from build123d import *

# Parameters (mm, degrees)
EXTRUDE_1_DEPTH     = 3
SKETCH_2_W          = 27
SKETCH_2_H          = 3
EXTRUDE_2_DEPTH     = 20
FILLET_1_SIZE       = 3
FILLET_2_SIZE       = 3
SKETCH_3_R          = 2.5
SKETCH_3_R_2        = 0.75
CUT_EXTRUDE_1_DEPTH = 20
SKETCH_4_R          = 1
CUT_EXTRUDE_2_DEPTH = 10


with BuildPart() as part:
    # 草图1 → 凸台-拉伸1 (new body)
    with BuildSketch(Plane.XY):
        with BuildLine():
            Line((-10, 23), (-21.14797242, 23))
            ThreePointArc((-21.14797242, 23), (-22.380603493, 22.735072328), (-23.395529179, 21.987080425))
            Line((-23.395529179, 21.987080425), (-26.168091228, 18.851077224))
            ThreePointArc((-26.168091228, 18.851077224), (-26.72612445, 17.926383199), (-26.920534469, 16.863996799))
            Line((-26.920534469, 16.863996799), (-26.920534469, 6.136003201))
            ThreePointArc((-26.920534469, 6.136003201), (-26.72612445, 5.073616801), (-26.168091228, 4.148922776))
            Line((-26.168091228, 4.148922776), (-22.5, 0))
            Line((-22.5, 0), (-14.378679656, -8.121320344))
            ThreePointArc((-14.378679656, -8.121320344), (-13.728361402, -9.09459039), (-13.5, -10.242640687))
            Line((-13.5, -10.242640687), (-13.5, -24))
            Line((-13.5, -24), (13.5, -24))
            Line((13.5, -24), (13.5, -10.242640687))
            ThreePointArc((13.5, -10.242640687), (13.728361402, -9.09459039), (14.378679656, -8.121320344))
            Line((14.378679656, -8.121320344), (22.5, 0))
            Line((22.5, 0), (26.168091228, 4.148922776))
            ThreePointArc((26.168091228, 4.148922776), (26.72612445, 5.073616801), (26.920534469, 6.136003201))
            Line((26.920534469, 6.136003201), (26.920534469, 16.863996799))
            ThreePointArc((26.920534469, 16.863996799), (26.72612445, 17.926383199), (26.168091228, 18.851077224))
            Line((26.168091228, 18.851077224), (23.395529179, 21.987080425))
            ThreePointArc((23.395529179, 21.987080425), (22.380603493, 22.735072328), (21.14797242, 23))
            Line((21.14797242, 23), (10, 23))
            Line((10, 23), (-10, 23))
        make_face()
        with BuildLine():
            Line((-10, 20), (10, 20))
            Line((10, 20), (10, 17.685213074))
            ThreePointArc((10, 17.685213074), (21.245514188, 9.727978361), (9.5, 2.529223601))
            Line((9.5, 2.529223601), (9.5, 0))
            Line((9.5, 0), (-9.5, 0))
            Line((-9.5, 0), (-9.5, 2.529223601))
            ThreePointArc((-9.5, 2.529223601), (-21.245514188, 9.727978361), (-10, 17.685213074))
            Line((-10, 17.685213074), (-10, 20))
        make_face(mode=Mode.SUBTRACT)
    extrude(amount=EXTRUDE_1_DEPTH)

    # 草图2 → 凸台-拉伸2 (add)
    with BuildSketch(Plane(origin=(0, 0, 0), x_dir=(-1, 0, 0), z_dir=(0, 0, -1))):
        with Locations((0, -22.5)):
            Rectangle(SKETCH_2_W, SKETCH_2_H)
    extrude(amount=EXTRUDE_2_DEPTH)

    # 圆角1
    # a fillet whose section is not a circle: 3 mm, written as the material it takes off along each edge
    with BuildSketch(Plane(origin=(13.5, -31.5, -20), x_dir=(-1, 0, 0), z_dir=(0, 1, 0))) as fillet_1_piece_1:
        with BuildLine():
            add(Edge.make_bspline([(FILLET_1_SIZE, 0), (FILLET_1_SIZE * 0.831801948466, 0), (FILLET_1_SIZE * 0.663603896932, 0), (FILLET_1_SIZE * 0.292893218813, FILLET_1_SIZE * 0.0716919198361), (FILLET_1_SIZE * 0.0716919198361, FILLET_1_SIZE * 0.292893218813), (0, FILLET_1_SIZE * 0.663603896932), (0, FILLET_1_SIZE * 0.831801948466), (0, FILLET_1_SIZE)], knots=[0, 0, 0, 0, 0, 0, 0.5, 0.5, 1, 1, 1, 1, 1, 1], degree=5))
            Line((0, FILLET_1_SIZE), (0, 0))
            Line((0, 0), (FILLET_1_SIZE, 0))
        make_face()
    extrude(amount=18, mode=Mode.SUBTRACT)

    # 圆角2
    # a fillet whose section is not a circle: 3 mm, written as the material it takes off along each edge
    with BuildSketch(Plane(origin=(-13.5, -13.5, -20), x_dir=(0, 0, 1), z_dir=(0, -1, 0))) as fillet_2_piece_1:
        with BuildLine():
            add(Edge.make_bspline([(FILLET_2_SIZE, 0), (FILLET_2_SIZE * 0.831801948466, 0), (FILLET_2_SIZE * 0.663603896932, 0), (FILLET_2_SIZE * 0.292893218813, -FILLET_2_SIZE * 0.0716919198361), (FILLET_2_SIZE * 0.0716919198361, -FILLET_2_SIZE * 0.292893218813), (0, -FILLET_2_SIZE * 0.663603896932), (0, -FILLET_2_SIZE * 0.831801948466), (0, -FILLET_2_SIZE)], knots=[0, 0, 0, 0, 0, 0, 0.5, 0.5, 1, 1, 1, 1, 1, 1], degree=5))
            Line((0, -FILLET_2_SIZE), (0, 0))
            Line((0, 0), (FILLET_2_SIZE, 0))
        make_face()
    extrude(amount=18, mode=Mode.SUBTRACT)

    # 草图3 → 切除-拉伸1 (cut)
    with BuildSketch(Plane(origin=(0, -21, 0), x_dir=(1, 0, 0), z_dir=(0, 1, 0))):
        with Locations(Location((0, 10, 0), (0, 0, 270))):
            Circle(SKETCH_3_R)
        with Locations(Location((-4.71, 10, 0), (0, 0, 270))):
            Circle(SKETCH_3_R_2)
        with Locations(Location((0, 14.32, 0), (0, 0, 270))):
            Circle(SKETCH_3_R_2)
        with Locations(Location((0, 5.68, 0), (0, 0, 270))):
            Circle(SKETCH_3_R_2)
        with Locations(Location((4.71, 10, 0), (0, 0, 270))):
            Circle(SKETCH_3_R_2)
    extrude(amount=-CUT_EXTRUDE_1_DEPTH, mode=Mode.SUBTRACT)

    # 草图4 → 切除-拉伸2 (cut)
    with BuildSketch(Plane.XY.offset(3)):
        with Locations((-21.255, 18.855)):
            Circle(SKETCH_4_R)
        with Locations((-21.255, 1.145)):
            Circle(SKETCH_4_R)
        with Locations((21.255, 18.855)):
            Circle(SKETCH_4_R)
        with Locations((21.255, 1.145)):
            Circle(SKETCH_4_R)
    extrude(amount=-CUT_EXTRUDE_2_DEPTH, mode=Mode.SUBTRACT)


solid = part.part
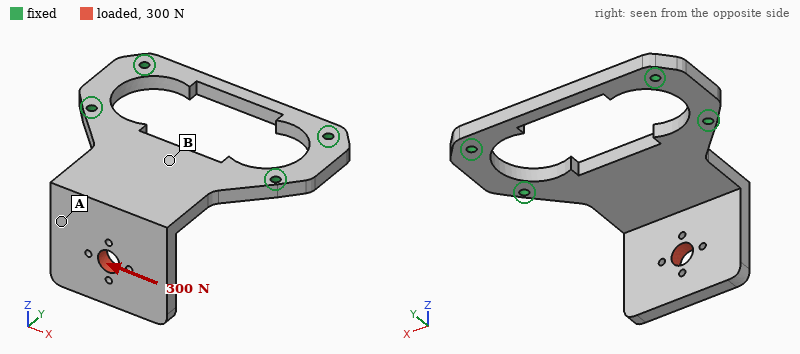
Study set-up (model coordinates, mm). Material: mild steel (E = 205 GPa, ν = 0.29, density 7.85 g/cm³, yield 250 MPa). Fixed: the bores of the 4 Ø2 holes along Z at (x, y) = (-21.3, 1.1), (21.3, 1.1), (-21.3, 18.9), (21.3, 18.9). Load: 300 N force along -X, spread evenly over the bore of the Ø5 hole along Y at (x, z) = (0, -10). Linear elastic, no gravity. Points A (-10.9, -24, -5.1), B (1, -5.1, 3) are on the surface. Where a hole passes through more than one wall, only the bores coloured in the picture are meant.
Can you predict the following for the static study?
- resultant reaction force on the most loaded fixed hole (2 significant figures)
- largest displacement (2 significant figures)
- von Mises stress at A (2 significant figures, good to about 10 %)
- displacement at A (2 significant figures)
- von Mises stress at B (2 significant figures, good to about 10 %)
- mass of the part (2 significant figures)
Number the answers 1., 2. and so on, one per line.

1. 260 N
2. 73 µm
3. 15 MPa
4. 38 µm
5. 43 MPa
6. 40 g
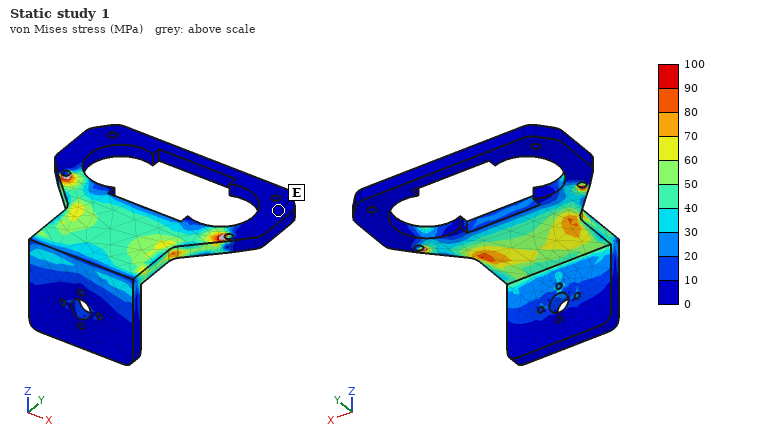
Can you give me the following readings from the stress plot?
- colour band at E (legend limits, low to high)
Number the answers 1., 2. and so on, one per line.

1. 0 to 10 MPa
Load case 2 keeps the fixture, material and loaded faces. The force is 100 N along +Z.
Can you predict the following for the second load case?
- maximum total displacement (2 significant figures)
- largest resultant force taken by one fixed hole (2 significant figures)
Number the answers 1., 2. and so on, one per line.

1. 0.14 mm
2. 57 N
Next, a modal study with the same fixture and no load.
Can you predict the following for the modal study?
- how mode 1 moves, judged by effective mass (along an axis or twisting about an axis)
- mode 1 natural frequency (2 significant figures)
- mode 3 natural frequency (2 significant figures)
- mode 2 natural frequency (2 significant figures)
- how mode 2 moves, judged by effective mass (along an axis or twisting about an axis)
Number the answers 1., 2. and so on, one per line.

1. along Z
2. 1100 Hz
3. 3800 Hz
4. 3100 Hz
5. along X
